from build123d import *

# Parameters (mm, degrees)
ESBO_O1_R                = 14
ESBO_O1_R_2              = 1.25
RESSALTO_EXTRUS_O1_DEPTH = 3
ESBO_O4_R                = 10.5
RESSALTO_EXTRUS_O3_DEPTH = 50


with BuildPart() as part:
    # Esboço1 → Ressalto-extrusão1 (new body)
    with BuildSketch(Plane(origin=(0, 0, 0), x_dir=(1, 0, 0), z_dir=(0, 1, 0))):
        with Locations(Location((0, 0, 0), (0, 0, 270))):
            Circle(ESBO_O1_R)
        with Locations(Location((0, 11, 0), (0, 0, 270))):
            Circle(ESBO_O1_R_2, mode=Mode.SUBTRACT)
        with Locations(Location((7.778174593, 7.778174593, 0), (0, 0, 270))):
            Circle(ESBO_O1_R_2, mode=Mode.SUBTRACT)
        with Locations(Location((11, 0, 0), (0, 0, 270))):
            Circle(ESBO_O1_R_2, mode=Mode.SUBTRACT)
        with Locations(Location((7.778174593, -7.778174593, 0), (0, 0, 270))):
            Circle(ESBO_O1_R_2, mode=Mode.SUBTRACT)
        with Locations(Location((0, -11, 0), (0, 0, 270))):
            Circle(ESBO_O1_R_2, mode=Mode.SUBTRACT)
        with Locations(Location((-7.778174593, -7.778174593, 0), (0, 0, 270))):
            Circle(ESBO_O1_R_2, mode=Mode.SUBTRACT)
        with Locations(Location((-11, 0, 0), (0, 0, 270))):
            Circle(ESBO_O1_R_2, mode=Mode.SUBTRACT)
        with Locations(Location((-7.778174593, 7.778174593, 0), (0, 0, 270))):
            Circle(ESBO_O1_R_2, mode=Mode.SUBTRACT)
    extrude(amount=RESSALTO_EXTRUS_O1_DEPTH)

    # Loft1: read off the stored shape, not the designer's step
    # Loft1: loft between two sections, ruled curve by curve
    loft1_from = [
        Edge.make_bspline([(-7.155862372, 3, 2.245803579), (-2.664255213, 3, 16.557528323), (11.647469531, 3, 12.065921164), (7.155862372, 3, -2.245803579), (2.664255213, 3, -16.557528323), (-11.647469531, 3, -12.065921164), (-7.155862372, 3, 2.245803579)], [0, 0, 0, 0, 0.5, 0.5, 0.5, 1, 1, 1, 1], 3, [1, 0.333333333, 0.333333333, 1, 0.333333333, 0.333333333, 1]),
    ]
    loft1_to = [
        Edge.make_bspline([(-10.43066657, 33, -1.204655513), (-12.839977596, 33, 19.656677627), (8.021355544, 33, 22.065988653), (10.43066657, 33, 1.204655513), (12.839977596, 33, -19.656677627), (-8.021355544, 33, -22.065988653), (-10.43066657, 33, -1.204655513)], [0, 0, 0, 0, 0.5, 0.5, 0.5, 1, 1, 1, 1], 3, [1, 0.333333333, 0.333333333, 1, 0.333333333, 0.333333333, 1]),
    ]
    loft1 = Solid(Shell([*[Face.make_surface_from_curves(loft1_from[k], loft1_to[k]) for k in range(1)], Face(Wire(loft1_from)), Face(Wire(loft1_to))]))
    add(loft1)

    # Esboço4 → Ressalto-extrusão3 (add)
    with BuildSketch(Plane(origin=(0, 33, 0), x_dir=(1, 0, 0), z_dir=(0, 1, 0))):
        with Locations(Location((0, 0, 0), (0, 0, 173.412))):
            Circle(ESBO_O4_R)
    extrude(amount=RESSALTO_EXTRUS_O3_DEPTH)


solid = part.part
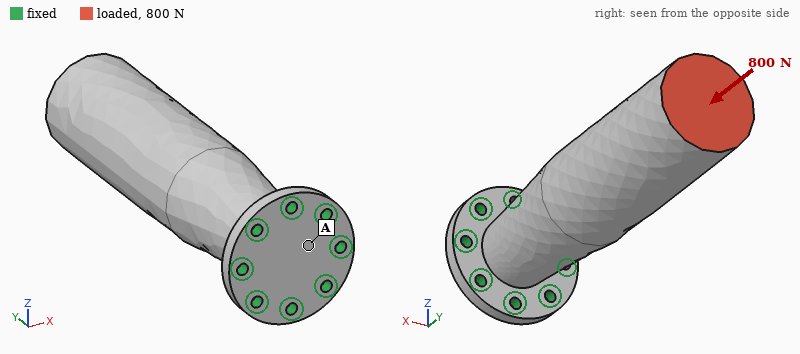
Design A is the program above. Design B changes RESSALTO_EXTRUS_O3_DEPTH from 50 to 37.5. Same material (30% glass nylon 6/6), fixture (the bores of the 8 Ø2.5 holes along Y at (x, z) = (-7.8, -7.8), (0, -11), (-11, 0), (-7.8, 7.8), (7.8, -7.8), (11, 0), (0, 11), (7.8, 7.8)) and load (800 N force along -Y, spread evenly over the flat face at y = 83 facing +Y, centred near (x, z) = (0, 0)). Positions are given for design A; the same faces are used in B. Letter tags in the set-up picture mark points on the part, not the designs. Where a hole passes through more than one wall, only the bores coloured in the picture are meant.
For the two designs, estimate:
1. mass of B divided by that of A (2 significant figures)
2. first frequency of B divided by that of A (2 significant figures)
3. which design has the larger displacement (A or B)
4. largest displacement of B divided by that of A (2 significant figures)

0.84
1.3
A
0.91
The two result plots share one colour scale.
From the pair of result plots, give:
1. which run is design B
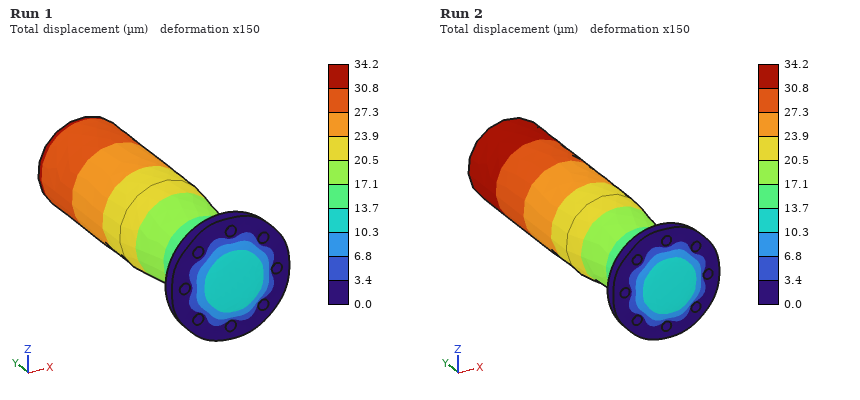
Run 1
